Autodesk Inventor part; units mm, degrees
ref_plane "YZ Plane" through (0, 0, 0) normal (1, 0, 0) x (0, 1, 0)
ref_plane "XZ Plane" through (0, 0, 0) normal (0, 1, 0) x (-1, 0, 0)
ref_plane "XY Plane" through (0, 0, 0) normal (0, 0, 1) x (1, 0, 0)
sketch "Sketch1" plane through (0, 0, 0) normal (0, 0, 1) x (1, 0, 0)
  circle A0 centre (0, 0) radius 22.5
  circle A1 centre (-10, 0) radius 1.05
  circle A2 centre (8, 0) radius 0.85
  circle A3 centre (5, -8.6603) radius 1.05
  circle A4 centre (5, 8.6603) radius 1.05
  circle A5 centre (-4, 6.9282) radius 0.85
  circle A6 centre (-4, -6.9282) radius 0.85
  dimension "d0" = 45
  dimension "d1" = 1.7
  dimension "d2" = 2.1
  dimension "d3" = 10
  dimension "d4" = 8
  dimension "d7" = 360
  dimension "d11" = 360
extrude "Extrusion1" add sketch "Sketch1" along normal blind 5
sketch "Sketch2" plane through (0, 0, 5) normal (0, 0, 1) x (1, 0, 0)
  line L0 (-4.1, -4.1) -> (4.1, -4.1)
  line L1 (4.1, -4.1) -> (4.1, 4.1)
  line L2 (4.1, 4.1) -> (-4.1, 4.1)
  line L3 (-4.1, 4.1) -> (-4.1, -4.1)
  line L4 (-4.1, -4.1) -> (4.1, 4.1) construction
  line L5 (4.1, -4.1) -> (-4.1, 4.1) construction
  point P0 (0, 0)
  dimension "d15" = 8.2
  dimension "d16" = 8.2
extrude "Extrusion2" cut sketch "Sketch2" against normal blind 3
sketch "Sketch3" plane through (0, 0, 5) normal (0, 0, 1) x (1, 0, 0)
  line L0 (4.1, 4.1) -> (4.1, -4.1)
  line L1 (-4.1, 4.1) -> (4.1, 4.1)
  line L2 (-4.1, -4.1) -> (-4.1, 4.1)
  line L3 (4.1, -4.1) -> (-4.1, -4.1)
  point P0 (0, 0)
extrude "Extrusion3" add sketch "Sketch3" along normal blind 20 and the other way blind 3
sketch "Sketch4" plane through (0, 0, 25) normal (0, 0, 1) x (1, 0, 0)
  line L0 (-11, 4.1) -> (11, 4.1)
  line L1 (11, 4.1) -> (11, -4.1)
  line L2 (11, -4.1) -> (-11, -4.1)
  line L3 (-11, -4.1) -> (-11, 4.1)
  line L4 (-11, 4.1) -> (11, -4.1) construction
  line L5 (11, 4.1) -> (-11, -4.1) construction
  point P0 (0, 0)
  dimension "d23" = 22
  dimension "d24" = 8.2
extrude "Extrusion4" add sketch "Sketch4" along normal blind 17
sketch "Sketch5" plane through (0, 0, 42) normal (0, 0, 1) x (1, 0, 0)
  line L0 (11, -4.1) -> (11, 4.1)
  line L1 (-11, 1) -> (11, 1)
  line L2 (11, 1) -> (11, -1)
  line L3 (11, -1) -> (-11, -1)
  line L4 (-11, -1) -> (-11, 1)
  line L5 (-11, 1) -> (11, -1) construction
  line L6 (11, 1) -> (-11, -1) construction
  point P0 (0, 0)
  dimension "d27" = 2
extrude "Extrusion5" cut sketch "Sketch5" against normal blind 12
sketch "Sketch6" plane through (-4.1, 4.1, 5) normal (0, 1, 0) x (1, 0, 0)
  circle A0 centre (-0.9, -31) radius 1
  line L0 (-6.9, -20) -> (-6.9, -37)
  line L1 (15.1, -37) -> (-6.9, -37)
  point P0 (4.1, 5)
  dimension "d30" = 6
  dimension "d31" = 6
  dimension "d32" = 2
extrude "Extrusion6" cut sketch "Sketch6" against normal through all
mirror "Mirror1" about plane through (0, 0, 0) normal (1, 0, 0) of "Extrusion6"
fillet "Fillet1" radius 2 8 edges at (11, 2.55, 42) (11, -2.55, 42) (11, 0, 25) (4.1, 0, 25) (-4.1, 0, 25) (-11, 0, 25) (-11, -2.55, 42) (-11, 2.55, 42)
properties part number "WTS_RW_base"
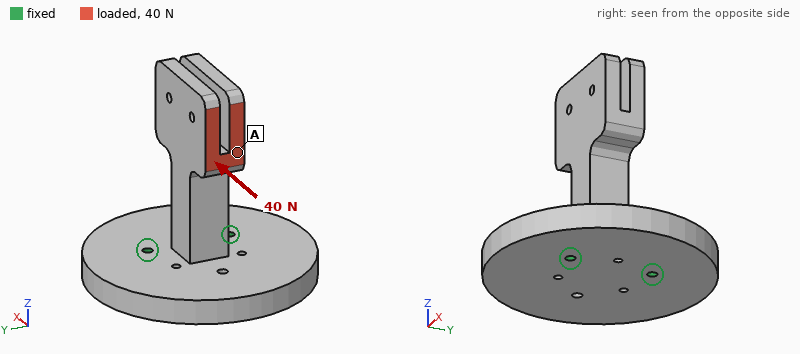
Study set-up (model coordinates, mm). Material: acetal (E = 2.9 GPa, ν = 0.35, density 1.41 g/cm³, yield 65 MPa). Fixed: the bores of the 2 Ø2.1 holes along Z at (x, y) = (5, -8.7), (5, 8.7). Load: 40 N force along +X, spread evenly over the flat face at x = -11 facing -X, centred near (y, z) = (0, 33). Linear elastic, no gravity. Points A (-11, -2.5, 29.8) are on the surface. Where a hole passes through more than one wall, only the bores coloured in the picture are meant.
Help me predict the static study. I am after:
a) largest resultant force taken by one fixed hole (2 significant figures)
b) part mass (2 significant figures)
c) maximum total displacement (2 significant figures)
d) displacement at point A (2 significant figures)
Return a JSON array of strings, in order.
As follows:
["21 N", "16 g", "0.83 mm", "0.58 mm"]
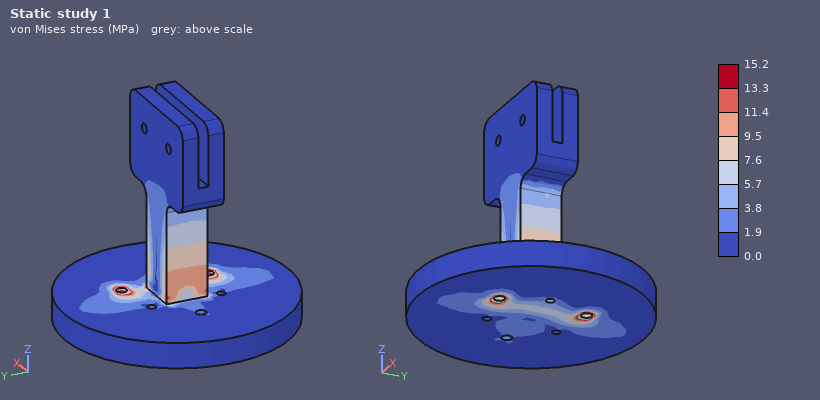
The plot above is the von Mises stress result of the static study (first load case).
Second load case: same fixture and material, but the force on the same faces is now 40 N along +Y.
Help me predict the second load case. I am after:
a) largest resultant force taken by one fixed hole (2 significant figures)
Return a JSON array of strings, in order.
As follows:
["84 N"]
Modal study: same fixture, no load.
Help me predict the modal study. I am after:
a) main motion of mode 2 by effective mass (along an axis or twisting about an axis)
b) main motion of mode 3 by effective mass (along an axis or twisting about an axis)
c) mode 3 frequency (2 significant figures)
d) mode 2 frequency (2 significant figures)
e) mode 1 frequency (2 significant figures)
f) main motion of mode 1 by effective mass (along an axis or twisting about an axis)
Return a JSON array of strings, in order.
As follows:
["along Y", "along Z", "1800 Hz", "800 Hz", "630 Hz", "along X"]
